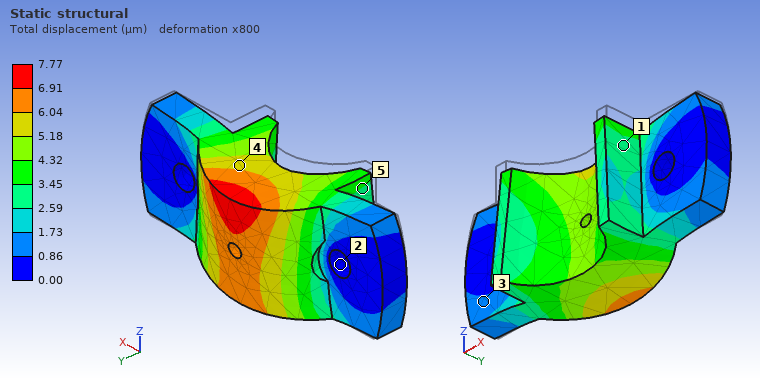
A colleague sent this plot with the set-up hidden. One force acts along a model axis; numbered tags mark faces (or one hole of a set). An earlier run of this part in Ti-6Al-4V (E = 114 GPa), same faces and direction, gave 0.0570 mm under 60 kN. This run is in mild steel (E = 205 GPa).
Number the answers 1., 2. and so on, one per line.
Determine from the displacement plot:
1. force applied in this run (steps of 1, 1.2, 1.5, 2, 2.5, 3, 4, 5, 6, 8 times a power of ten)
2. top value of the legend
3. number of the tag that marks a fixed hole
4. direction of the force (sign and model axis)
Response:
1. 15 kN
2. 7.77 µm
3. 2
4. -Z
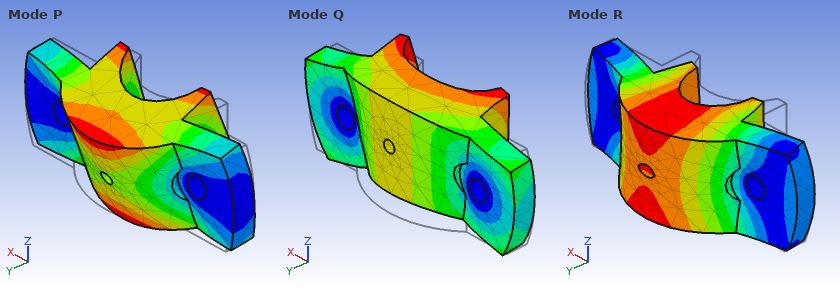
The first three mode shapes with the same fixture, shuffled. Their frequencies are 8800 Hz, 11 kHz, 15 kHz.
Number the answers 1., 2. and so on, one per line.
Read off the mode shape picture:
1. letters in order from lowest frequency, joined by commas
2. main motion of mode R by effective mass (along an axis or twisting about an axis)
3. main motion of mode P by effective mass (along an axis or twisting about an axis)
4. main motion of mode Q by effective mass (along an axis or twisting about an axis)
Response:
1. P, R, Q
2. along Y
3. twisting about X
4. along Z
